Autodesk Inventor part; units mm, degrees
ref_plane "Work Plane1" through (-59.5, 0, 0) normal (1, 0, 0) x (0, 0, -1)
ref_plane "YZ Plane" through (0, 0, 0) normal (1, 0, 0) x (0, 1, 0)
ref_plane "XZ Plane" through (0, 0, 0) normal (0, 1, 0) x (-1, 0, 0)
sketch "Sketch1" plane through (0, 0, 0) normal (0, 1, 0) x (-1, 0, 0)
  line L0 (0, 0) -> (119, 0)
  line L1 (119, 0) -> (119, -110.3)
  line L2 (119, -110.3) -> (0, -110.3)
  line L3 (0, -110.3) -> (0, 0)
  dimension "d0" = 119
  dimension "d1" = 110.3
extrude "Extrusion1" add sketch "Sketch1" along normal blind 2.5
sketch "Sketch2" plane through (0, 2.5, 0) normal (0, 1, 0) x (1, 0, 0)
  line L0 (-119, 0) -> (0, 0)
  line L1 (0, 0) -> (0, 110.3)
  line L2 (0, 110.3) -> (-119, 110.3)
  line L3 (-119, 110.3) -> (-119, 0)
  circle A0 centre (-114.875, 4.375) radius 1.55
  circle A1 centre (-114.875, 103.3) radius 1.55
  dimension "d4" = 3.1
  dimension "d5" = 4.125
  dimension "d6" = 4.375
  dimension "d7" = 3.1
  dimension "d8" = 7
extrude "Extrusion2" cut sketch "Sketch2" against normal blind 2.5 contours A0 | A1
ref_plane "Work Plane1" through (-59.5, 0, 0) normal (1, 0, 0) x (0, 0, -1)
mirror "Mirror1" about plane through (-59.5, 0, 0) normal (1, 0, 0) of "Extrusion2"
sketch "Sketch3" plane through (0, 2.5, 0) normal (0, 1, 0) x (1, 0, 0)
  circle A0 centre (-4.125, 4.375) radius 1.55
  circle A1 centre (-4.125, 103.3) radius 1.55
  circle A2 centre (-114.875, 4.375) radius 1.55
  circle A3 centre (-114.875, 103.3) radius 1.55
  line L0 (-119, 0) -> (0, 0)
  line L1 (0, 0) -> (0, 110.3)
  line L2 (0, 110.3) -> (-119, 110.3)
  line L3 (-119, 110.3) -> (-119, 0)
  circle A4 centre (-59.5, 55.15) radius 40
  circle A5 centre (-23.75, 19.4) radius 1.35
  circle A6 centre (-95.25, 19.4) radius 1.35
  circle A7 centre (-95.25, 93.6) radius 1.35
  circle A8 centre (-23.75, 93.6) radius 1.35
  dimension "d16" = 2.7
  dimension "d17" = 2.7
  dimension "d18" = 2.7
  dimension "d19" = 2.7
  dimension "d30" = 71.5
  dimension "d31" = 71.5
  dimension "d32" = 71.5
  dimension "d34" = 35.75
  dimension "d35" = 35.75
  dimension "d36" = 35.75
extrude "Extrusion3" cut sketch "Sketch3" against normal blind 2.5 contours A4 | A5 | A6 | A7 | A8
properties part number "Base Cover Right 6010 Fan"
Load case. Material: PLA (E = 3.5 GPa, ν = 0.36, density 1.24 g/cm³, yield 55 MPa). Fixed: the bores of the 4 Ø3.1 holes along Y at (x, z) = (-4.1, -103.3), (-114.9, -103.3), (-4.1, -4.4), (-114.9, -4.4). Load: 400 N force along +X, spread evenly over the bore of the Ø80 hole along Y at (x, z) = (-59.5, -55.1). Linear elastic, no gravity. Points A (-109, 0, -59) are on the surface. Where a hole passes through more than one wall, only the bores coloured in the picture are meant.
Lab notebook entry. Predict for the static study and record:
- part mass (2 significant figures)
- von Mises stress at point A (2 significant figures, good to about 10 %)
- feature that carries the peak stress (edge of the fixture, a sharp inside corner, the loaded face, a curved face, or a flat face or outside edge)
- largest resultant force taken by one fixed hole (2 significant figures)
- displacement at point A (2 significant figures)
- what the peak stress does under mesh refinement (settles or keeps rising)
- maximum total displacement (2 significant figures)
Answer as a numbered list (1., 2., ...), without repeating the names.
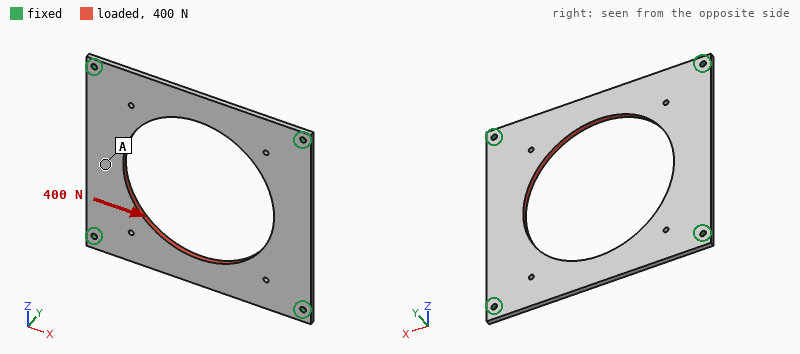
1. 25 g
2. 0.64 MPa
3. edge of the fixture
4. 110 N
5. 75 µm
6. keeps rising
7. 76 µm
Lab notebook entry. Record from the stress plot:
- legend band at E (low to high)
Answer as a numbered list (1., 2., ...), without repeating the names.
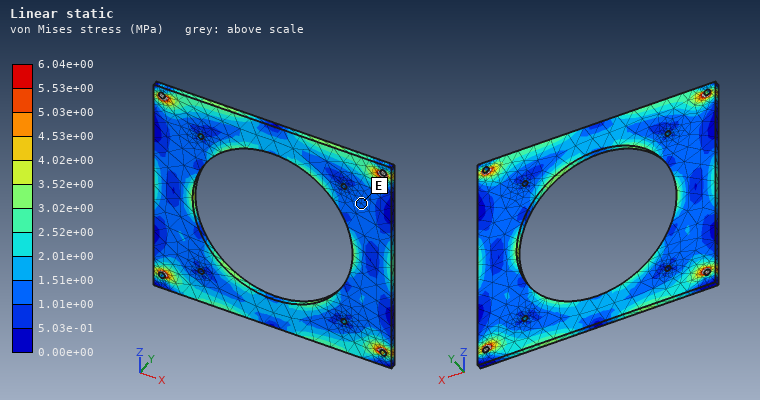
1. 1.01e+00 to 1.51e+00 MPa
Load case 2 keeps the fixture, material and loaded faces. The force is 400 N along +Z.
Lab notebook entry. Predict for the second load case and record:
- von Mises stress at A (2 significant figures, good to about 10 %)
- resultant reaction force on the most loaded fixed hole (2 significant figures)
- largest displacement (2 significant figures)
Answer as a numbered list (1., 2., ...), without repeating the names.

1. 2.4 MPa
2. 110 N
3. 0.10 mm
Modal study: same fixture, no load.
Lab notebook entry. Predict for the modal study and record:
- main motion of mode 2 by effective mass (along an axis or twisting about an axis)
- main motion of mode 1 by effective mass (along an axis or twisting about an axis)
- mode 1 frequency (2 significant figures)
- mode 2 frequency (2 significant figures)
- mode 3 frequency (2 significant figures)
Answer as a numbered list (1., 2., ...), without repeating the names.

1. twisting about X
2. along Y
3. 320 Hz
4. 390 Hz
5. 420 Hz
